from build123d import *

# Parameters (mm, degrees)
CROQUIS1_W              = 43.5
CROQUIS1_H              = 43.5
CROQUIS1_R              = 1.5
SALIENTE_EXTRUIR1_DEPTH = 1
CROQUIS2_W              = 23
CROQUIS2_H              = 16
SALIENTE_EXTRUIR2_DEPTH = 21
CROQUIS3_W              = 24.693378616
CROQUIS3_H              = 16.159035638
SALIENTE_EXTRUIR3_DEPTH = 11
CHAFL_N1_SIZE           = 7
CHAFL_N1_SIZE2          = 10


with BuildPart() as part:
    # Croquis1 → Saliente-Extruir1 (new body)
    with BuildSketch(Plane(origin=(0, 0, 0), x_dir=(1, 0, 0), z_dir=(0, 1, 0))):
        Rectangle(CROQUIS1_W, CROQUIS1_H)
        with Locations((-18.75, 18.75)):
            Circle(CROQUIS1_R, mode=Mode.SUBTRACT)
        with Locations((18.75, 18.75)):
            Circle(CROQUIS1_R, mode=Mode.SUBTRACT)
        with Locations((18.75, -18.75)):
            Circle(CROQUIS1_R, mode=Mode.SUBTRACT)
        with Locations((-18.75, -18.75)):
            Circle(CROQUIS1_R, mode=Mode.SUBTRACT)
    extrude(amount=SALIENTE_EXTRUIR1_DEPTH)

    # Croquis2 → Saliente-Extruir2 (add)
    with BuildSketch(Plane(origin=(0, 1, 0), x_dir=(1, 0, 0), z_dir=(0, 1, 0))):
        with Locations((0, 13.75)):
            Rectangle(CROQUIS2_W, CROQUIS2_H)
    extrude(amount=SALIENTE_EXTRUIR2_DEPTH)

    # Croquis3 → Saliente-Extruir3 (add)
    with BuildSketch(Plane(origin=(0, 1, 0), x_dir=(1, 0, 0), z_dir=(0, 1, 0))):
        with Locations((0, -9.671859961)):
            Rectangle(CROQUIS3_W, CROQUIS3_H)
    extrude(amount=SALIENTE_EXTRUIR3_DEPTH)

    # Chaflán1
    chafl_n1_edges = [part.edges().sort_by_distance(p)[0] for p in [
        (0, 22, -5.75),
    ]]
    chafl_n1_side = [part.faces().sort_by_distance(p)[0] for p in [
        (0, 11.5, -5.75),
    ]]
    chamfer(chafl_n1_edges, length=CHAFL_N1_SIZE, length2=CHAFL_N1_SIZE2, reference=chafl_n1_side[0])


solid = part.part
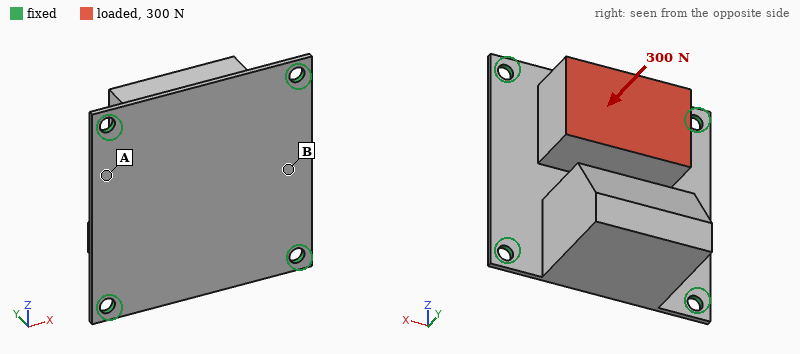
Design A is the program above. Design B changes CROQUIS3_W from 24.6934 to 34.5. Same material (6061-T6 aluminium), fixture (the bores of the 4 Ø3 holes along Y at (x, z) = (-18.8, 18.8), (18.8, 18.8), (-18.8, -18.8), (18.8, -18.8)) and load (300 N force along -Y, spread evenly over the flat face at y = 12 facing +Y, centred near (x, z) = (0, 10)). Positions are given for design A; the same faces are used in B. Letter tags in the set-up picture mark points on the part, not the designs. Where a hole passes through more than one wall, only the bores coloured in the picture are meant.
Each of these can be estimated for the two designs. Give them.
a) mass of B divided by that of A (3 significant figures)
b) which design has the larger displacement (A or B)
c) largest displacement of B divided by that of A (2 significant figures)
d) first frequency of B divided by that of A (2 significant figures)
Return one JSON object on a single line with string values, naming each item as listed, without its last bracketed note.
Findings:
{"mass of B divided by that of A": "1.13", "which design has the larger displacement": "A", "largest displacement of B divided by that of A": "0.78", "first frequency of B divided by that of A": "1.0"}
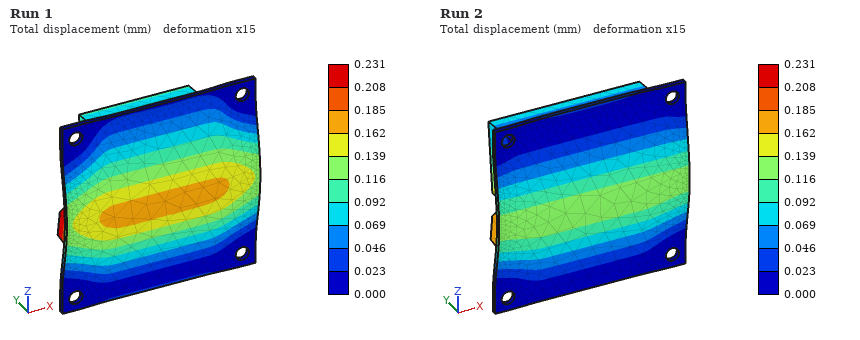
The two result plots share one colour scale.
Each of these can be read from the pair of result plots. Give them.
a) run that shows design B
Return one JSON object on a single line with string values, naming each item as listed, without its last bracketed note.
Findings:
{"run that shows design B": "Run 2"}
